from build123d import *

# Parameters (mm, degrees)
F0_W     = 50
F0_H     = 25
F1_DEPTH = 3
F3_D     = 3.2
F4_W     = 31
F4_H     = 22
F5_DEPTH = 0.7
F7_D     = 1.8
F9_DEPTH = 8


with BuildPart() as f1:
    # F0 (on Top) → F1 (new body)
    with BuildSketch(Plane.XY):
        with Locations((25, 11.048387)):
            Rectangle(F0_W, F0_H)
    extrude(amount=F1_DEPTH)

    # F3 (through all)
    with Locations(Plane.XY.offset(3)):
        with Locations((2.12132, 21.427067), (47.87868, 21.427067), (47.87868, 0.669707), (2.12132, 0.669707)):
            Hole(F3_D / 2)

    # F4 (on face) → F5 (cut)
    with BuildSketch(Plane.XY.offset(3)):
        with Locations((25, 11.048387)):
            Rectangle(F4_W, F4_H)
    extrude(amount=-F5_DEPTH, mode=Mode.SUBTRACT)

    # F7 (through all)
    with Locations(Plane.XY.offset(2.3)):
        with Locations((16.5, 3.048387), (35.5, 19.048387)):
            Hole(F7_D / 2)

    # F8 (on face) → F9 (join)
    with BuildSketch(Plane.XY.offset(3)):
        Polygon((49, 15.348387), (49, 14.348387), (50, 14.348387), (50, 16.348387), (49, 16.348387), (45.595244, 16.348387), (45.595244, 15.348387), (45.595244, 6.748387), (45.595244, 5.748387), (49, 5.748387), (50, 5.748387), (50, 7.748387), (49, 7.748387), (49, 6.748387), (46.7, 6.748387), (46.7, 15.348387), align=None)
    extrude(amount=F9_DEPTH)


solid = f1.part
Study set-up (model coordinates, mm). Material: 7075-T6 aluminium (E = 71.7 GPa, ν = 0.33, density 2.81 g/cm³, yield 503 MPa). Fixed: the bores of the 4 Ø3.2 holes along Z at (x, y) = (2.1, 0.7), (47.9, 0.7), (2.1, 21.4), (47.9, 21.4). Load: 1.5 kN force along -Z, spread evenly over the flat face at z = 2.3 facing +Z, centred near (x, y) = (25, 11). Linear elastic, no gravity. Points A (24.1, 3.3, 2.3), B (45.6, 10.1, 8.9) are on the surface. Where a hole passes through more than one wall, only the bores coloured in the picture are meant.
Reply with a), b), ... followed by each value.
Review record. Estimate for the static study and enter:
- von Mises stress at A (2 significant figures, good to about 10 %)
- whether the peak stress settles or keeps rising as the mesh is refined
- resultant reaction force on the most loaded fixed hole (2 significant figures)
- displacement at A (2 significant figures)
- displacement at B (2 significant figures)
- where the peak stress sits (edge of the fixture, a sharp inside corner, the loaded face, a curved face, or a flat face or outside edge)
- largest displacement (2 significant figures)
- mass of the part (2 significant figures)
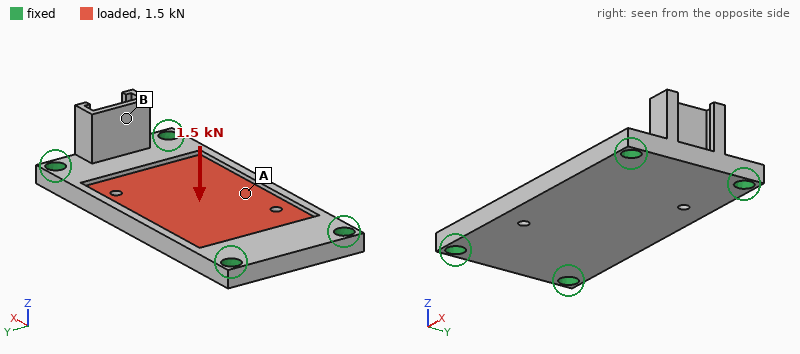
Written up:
a) 110 MPa
b) keeps rising
c) 460 N
d) 0.19 mm
e) 0.049 mm
f) edge of the fixture
g) 0.19 mm
h) 9.3 g
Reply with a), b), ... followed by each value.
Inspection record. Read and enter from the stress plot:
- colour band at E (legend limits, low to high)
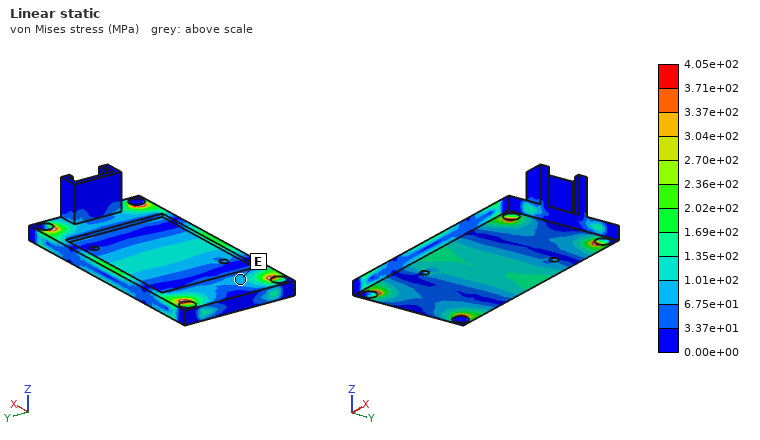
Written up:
a) 6.75e+01 to 1.01e+02 MPa
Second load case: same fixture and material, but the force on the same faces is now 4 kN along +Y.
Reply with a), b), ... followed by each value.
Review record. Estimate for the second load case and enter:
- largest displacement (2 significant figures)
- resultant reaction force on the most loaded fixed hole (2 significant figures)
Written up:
a) 68 µm
b) 1.3 kN
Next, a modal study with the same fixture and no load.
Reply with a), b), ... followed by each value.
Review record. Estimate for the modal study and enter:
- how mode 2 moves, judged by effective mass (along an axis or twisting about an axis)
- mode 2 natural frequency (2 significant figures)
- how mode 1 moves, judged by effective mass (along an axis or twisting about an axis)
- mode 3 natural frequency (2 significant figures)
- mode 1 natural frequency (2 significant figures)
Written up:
a) twisting about X
b) 11 kHz
c) along Z
d) 17 kHz
e) 6800 Hz
